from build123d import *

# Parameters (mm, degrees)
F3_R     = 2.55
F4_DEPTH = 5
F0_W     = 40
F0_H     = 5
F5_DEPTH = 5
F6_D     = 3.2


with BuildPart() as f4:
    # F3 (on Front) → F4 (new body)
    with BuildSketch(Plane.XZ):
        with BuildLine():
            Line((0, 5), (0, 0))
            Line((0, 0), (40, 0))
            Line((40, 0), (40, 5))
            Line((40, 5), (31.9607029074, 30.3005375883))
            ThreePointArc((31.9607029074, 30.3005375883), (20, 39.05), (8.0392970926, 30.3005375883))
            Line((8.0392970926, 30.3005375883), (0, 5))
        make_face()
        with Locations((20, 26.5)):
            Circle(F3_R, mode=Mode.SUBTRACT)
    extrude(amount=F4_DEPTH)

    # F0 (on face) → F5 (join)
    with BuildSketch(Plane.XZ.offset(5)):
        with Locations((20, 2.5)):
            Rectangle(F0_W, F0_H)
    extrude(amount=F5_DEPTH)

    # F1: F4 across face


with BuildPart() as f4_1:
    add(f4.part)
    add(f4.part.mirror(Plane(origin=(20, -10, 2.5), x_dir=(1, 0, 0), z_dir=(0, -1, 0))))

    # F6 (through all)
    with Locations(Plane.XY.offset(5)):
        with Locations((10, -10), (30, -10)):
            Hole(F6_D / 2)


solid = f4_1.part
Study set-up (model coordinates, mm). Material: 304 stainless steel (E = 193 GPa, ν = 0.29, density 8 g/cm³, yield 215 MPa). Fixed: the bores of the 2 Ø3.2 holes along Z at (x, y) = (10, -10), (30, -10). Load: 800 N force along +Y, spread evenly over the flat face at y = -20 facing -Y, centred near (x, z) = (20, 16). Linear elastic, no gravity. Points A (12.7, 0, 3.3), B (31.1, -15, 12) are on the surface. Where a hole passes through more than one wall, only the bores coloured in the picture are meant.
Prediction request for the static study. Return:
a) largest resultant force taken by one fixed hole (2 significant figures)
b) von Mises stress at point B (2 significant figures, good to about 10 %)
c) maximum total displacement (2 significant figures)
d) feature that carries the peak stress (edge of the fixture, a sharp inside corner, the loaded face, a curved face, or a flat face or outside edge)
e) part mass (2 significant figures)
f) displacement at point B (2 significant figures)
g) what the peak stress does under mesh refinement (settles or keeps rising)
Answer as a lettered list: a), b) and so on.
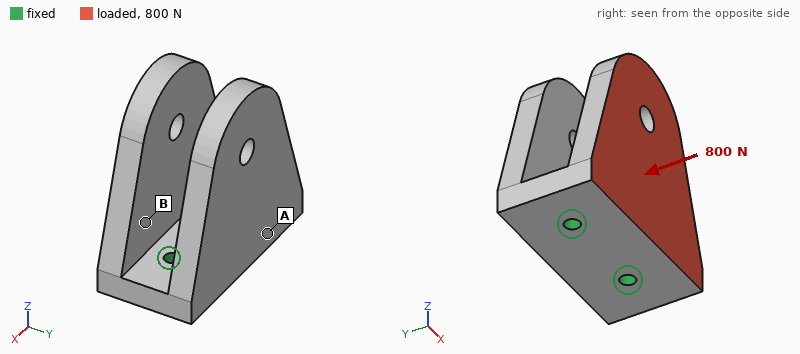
a) 400 N
b) 35 MPa
c) 83 µm
d) edge of the fixture
e) 110 g
f) 14 µm
g) keeps rising
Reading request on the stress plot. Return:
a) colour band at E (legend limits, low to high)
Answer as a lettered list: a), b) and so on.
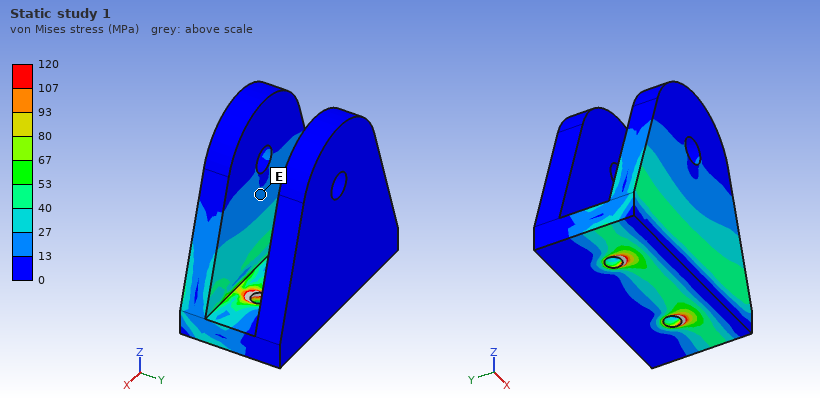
a) 13 to 27 MPa
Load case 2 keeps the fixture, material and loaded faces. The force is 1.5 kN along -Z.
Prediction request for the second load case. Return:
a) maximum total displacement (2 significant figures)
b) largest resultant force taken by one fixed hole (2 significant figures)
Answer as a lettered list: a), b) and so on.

a) 59 µm
b) 750 N
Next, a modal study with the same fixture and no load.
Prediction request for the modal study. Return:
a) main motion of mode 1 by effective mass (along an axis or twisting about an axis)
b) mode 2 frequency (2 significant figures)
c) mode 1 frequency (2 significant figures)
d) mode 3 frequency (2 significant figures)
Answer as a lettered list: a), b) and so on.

a) along Y
b) 3200 Hz
c) 2900 Hz
d) 7900 Hz
